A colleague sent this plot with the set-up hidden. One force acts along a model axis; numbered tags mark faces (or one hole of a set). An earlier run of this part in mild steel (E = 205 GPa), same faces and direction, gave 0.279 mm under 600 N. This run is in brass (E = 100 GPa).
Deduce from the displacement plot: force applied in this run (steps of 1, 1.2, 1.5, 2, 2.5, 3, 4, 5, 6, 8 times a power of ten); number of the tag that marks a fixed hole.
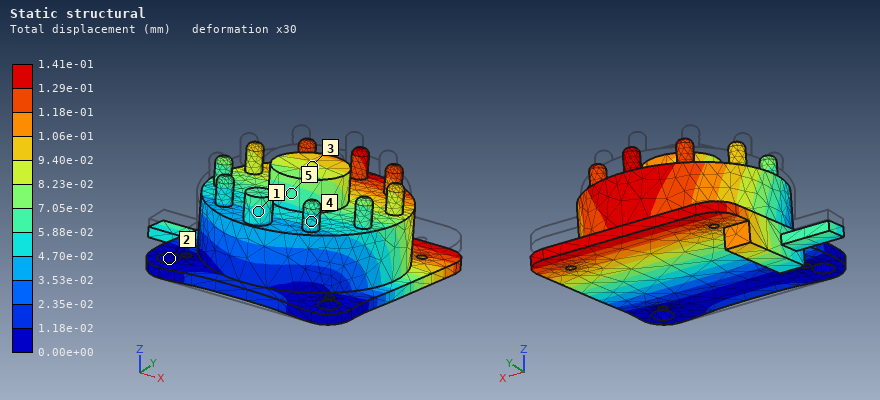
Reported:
150 N
2
